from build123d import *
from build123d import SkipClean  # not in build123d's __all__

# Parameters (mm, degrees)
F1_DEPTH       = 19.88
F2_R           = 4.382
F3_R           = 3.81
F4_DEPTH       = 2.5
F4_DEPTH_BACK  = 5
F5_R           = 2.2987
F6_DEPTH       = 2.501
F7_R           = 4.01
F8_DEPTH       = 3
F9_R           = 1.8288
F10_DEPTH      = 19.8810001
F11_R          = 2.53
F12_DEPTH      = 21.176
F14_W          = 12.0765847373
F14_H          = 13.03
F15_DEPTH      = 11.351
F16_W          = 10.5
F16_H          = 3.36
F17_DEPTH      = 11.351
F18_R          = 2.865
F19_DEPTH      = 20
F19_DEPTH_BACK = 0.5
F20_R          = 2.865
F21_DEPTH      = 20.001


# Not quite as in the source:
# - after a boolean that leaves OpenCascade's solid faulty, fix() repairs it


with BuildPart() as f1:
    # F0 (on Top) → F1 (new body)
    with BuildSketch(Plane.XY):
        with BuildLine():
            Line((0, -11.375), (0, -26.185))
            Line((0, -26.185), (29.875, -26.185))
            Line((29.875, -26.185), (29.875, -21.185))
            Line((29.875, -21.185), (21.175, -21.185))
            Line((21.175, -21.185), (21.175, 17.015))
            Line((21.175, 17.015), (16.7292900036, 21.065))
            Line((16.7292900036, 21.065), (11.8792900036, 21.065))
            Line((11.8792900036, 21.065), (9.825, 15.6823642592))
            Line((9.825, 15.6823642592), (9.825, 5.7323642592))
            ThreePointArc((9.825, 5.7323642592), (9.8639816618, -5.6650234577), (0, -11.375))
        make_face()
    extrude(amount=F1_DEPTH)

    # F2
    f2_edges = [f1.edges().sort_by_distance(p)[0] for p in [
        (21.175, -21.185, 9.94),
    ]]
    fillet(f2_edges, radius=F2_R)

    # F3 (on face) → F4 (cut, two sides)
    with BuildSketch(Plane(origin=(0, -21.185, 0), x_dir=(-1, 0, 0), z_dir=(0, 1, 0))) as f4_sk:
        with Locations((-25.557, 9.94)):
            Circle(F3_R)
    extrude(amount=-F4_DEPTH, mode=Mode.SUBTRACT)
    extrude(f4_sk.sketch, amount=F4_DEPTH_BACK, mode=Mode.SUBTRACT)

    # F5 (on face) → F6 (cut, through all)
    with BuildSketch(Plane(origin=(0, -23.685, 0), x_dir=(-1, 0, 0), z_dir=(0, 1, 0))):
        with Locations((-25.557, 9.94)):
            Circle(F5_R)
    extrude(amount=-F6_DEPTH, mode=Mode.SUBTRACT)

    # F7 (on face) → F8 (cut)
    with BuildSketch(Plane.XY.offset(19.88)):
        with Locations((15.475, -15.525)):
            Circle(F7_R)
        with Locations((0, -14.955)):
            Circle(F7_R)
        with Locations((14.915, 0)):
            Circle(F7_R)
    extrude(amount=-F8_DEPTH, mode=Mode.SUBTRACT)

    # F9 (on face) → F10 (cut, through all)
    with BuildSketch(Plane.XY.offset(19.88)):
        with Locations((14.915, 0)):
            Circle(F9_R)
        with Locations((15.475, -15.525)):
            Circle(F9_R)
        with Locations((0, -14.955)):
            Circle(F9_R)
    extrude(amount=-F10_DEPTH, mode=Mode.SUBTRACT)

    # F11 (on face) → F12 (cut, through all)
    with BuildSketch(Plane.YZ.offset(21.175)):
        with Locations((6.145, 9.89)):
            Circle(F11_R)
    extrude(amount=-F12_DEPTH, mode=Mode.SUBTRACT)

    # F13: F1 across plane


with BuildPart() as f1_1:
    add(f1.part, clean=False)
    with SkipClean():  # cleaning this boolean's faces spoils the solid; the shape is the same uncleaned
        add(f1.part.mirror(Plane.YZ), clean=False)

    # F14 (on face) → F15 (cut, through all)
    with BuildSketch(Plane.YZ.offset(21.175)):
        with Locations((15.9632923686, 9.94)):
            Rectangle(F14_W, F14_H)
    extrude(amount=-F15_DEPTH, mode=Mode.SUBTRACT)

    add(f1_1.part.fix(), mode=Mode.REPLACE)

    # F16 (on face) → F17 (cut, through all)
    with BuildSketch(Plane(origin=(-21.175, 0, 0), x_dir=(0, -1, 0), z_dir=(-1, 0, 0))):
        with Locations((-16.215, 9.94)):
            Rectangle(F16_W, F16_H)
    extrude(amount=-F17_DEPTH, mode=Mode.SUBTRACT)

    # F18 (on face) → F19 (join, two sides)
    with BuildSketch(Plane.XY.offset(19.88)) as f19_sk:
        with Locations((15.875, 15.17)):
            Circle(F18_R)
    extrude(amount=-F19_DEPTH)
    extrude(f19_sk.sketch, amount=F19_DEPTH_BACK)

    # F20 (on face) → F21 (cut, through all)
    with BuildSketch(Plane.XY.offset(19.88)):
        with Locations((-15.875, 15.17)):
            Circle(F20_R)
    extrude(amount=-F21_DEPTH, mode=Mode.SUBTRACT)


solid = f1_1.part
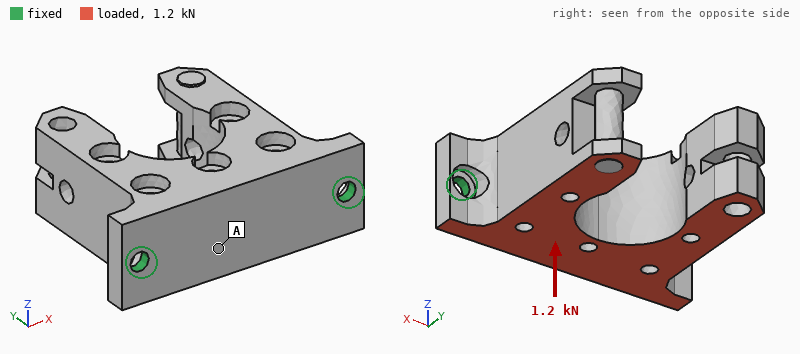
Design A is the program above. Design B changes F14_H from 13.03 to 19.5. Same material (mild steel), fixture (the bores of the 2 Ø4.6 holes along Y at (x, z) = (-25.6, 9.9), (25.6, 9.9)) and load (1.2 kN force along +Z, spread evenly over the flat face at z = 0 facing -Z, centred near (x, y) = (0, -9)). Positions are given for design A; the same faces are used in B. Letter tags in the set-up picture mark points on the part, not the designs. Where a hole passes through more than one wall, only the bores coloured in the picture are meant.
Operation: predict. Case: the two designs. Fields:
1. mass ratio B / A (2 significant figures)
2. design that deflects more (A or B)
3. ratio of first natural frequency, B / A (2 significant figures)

0.98
B
1.0
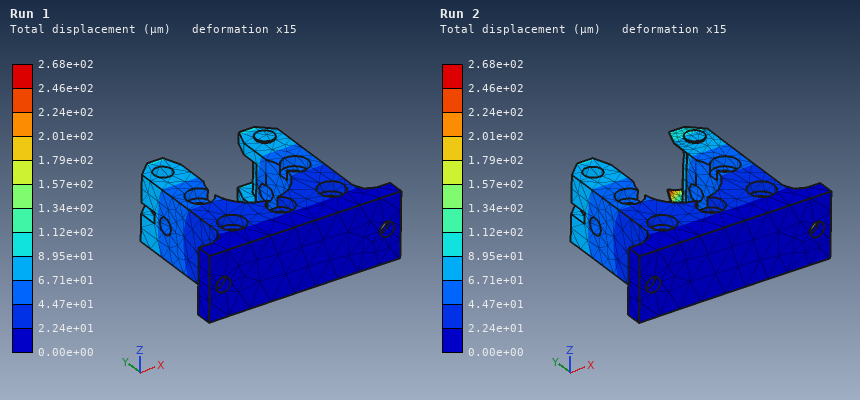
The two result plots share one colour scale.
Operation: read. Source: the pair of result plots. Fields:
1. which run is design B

Run 2
